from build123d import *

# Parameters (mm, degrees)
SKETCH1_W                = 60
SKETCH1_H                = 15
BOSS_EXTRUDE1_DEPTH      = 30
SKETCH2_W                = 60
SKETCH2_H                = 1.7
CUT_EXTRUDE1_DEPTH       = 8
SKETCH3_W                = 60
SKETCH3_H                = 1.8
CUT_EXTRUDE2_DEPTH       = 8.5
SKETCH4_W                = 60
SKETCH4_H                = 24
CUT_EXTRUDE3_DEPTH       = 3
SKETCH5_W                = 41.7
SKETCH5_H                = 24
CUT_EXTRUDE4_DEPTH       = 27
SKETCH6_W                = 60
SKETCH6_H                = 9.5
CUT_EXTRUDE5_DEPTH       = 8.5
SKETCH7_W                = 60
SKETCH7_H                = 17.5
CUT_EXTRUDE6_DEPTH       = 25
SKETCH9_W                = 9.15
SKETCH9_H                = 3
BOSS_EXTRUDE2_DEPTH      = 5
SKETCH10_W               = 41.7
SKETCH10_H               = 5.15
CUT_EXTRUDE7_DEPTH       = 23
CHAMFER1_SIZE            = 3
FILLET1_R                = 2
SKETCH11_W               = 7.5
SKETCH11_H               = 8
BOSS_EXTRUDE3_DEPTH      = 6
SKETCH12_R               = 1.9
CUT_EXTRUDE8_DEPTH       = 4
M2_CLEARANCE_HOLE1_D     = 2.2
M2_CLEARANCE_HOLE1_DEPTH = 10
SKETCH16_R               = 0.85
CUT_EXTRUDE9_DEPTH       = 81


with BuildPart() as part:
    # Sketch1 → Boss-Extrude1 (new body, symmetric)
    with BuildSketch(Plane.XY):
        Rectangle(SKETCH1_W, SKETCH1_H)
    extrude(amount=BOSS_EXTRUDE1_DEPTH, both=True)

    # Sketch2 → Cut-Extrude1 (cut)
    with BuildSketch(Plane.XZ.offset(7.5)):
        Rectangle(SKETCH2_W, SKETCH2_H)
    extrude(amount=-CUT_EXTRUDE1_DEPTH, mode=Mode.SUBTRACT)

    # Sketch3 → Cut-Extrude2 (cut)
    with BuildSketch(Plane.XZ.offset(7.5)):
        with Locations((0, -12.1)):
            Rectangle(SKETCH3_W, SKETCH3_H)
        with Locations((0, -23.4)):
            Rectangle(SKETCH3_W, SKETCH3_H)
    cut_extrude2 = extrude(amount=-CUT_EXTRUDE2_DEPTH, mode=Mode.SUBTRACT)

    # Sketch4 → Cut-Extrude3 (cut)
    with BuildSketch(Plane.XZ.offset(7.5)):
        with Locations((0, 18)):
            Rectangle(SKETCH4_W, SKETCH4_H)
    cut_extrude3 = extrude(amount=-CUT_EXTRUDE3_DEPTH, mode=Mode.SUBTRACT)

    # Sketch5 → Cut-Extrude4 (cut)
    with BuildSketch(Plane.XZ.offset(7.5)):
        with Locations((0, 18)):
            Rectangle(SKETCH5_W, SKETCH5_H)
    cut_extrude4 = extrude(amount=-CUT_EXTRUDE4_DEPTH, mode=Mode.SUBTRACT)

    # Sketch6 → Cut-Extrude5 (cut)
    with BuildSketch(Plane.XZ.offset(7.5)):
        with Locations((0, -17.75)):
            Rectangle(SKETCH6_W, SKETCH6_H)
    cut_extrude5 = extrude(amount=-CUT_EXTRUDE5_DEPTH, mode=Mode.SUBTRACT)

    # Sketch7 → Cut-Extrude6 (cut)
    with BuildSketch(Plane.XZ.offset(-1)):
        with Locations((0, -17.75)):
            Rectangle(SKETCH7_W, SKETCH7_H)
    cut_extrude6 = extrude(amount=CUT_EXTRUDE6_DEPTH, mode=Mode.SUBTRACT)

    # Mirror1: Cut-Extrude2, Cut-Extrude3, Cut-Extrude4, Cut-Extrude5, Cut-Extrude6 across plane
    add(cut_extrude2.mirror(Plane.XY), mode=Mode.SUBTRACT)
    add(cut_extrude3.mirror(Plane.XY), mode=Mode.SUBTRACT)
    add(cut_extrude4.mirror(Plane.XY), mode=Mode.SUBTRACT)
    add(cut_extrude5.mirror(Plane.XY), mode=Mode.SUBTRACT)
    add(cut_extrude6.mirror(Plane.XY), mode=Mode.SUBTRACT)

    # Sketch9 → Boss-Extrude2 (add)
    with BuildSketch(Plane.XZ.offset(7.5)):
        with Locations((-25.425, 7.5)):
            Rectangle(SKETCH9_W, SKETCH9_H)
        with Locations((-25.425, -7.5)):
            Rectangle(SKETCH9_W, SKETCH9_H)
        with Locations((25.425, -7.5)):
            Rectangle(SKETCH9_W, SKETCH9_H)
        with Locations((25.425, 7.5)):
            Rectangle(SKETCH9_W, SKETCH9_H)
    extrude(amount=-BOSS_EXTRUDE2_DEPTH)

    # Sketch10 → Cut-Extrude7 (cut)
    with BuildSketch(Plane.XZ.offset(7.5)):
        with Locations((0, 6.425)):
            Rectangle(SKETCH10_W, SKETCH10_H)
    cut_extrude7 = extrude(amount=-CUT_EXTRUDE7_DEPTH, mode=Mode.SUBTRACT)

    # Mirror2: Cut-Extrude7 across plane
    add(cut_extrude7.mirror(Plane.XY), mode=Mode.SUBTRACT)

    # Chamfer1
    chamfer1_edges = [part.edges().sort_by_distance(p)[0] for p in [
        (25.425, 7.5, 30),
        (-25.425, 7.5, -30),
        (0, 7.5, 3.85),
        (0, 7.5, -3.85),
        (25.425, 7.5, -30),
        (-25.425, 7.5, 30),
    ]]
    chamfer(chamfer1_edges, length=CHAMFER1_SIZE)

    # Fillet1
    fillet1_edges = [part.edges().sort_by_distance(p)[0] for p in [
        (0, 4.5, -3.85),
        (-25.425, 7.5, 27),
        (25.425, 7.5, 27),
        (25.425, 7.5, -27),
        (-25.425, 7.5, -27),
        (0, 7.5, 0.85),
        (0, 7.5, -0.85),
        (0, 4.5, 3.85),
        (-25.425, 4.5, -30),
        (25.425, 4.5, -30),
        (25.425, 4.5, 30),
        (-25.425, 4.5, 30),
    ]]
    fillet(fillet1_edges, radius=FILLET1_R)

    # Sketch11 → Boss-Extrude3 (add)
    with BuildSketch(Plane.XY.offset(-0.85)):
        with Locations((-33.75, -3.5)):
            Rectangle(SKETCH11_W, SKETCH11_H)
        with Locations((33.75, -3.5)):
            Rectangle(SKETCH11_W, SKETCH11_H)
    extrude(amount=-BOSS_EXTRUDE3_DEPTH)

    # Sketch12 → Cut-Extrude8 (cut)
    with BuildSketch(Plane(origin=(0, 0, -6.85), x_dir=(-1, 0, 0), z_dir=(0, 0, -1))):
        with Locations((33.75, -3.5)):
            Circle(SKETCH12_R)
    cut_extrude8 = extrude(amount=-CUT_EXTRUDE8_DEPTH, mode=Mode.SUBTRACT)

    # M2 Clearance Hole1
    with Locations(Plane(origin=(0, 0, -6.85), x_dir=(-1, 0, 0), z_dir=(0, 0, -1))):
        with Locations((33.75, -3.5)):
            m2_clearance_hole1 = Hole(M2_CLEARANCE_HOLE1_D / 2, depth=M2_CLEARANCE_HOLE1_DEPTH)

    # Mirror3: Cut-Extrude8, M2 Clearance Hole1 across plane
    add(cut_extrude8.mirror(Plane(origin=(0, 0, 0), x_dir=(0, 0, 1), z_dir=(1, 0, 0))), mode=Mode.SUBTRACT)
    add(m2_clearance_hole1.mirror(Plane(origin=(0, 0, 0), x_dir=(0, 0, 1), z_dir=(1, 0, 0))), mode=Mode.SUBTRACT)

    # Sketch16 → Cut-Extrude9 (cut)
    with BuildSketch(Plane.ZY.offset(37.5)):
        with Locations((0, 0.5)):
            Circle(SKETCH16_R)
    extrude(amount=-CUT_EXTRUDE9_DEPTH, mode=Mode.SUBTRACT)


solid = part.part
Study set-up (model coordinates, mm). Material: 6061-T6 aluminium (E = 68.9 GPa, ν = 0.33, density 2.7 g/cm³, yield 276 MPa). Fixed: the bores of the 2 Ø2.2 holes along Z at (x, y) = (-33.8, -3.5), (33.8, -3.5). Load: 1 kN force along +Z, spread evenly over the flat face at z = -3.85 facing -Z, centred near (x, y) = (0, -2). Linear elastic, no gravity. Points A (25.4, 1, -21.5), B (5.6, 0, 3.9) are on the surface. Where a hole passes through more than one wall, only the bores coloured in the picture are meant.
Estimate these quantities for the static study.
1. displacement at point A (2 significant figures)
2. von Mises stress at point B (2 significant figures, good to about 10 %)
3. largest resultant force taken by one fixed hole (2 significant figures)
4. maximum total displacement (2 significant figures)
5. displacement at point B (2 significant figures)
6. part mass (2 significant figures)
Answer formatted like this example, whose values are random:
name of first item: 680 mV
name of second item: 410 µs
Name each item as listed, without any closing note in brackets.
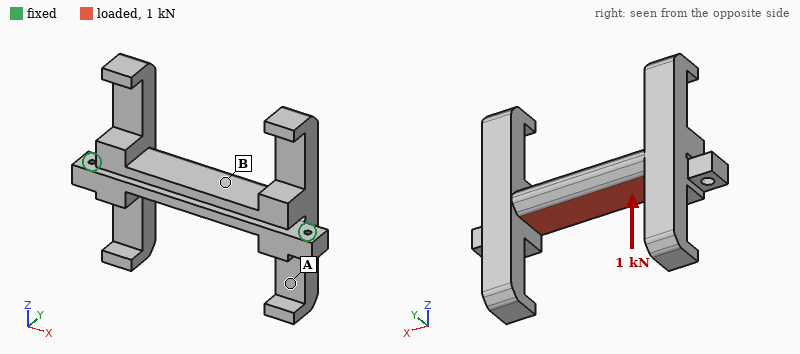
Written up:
displacement at point A: 0.13 mm
von Mises stress at point B: 73 MPa
largest resultant force taken by one fixed hole: 650 N
maximum total displacement: 0.19 mm
displacement at point B: 0.15 mm
part mass: 39 g
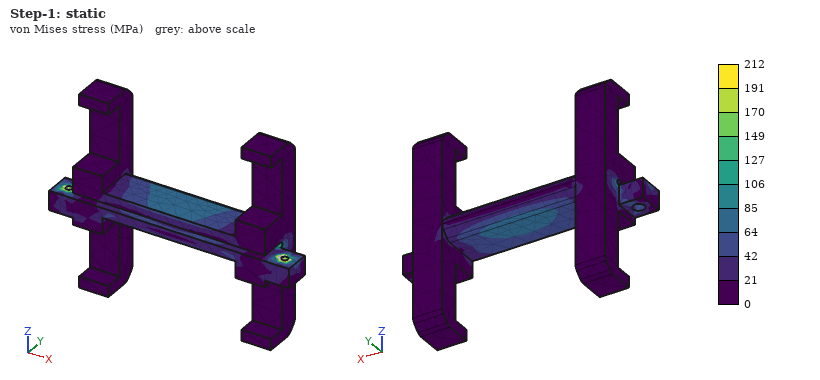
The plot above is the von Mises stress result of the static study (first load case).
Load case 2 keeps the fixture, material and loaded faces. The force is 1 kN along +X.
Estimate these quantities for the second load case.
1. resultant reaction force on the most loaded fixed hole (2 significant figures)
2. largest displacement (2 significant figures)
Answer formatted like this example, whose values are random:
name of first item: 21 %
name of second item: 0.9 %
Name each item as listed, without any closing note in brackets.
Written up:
resultant reaction force on the most loaded fixed hole: 500 N
largest displacement: 10 µm
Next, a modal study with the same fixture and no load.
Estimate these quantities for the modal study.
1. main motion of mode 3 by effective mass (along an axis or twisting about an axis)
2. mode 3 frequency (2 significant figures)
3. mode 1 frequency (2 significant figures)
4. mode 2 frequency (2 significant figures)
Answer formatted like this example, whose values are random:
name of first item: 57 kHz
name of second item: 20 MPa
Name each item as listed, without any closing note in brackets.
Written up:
main motion of mode 3 by effective mass: along Z
mode 3 frequency: 2600 Hz
mode 1 frequency: 1500 Hz
mode 2 frequency: 2300 Hz
